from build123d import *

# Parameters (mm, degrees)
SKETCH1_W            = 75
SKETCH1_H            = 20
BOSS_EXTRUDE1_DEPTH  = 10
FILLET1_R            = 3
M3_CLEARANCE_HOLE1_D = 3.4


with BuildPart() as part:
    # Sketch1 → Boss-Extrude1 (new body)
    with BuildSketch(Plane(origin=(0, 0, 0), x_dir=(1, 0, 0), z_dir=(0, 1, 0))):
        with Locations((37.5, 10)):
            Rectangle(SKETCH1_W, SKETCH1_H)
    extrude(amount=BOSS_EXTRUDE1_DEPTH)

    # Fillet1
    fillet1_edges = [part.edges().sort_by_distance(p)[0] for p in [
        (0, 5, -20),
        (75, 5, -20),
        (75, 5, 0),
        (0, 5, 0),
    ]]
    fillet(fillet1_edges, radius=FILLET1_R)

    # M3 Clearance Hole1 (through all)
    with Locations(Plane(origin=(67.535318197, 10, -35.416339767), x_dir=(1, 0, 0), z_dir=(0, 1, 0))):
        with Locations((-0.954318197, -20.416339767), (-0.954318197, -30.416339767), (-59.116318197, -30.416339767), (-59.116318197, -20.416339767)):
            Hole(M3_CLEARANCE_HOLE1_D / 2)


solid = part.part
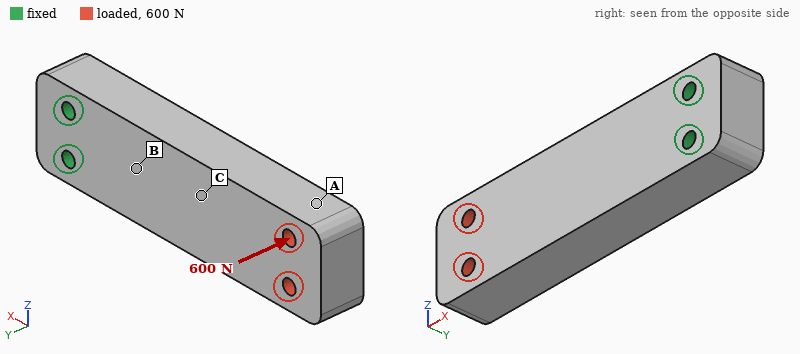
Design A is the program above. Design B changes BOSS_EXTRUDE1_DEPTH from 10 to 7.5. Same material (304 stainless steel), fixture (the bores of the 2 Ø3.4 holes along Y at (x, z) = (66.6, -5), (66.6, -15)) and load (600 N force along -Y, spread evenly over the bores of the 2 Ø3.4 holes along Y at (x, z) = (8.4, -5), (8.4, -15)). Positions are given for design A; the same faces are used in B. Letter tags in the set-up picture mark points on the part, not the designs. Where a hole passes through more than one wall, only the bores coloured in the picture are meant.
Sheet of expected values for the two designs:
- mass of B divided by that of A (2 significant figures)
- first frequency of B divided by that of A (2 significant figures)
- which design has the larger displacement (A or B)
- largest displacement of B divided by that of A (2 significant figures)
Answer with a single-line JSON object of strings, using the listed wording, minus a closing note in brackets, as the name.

{"mass of B divided by that of A": "0.75", "first frequency of B divided by that of A": "0.76", "which design has the larger displacement": "B", "largest displacement of B divided by that of A": "2.3"}
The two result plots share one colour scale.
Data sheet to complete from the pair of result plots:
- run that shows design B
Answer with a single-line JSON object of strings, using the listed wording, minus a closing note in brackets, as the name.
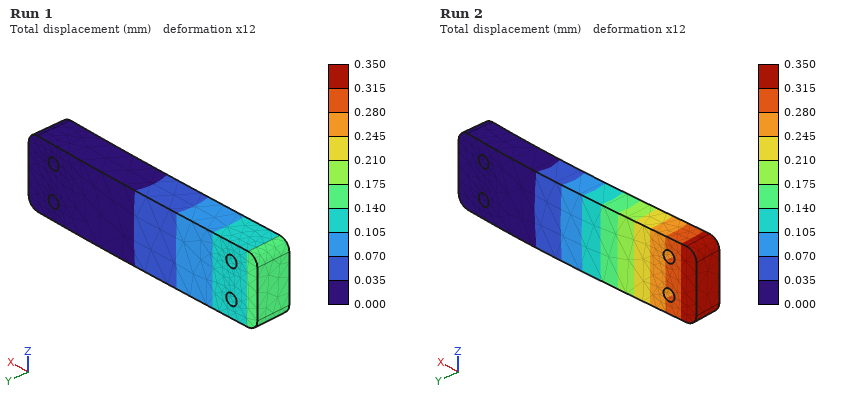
{"run that shows design B": "Run 2"}
